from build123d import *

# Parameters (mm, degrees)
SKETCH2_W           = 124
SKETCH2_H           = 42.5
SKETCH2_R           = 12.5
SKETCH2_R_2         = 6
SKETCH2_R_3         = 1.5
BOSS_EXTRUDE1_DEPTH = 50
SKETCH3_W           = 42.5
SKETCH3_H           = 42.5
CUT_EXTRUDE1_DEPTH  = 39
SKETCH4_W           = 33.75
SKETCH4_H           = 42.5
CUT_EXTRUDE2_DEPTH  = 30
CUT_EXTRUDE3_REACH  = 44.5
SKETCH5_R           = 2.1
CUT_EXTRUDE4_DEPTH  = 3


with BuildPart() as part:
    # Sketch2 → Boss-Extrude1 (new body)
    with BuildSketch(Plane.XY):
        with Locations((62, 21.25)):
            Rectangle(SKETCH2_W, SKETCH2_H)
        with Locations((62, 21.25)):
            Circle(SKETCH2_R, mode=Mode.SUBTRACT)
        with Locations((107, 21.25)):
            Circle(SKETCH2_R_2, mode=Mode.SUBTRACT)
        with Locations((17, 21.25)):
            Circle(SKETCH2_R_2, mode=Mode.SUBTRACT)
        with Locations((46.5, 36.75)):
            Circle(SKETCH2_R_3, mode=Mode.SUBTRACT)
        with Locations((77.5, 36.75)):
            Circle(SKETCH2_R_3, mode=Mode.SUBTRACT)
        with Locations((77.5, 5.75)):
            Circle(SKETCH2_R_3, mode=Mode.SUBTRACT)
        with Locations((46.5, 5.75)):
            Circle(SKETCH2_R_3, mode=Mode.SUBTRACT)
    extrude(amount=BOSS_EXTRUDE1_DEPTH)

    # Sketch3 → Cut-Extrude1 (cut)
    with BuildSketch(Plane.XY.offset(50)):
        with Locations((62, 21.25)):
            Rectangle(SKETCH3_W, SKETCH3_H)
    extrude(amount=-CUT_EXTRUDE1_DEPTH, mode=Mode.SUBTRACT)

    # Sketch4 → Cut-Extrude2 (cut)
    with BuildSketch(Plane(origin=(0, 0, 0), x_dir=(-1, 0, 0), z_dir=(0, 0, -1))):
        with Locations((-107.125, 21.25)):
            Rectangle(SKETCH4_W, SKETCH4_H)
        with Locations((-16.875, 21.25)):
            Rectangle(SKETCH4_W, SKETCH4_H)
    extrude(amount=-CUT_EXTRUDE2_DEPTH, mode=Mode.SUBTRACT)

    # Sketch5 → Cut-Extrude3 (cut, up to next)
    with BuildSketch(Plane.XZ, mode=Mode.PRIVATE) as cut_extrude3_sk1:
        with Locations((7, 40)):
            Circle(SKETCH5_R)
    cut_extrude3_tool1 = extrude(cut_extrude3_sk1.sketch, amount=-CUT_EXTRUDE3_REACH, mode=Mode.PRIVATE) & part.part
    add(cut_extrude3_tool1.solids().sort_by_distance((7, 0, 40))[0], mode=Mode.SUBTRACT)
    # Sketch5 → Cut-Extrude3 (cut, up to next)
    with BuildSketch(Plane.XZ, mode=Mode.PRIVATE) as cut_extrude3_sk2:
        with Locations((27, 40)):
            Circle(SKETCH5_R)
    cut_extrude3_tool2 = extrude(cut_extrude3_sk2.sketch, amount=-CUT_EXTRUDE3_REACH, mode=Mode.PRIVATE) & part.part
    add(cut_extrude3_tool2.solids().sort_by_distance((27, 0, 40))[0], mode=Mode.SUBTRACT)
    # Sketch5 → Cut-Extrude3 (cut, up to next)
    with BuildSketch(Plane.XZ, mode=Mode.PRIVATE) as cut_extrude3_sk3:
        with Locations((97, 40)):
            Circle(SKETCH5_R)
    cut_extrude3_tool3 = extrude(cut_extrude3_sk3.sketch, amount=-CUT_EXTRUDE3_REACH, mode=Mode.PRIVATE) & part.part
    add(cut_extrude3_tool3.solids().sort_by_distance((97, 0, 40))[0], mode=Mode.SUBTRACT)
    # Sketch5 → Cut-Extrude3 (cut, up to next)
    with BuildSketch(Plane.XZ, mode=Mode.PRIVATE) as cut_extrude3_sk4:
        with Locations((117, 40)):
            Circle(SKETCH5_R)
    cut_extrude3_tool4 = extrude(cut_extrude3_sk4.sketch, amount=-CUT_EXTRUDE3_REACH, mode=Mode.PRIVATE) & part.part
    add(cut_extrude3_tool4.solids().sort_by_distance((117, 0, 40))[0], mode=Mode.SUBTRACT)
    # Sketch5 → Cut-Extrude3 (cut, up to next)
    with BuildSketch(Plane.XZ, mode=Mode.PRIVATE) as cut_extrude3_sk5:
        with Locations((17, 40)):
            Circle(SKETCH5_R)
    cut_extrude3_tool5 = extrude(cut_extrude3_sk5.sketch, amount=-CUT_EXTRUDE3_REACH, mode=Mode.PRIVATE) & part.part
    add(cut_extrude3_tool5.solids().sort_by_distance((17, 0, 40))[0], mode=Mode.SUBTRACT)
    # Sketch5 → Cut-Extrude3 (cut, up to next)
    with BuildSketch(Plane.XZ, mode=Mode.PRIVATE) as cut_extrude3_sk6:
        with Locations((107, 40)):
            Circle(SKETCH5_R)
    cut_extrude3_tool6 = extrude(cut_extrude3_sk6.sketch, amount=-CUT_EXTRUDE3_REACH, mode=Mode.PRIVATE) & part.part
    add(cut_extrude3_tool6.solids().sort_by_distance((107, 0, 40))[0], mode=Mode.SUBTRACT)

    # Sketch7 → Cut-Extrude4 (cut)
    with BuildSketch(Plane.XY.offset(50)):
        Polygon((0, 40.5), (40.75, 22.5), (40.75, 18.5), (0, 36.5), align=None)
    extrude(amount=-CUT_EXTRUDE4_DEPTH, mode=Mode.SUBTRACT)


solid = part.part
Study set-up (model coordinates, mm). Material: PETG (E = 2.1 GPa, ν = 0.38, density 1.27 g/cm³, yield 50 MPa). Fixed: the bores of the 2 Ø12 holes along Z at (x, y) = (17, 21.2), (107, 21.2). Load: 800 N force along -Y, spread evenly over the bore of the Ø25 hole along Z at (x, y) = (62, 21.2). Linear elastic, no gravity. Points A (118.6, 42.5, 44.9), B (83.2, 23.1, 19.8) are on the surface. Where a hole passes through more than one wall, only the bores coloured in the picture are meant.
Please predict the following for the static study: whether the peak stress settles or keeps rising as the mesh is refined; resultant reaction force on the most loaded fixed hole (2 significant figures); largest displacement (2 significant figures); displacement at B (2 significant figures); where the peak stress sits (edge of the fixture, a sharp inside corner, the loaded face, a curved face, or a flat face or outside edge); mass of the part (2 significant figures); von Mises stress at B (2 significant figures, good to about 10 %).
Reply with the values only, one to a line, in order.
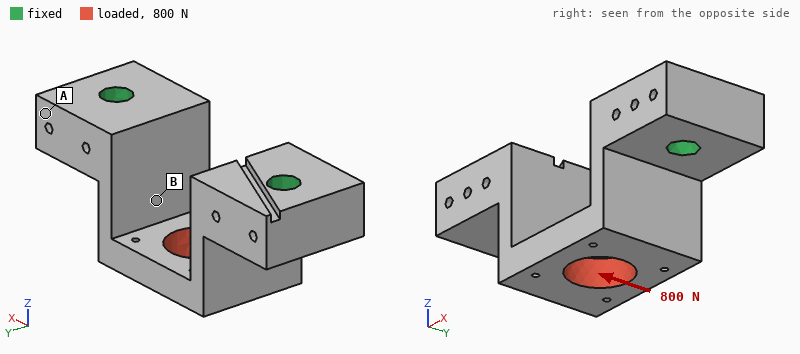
keeps rising
400 N
0.37 mm
0.15 mm
edge of the fixture
120 g
3.5 MPa
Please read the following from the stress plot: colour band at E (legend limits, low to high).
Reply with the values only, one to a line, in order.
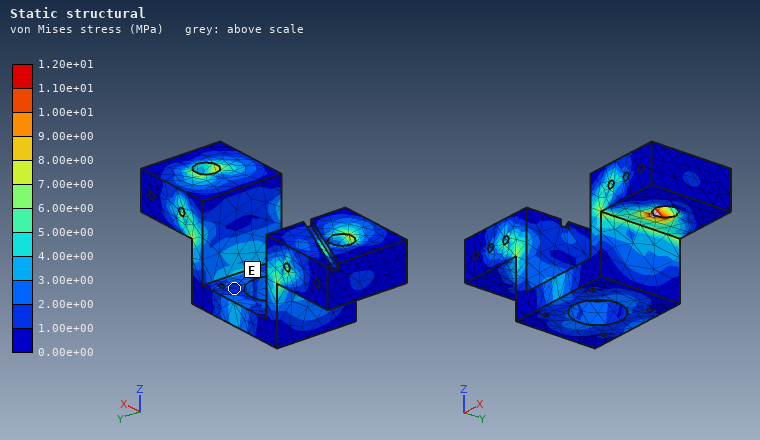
1.00e+00 to 2.00e+00 MPa
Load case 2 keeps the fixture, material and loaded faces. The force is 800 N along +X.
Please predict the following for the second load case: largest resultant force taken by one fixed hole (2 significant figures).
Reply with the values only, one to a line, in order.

460 N
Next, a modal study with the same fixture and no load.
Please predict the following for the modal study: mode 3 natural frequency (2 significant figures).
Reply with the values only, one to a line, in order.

1900 Hz
